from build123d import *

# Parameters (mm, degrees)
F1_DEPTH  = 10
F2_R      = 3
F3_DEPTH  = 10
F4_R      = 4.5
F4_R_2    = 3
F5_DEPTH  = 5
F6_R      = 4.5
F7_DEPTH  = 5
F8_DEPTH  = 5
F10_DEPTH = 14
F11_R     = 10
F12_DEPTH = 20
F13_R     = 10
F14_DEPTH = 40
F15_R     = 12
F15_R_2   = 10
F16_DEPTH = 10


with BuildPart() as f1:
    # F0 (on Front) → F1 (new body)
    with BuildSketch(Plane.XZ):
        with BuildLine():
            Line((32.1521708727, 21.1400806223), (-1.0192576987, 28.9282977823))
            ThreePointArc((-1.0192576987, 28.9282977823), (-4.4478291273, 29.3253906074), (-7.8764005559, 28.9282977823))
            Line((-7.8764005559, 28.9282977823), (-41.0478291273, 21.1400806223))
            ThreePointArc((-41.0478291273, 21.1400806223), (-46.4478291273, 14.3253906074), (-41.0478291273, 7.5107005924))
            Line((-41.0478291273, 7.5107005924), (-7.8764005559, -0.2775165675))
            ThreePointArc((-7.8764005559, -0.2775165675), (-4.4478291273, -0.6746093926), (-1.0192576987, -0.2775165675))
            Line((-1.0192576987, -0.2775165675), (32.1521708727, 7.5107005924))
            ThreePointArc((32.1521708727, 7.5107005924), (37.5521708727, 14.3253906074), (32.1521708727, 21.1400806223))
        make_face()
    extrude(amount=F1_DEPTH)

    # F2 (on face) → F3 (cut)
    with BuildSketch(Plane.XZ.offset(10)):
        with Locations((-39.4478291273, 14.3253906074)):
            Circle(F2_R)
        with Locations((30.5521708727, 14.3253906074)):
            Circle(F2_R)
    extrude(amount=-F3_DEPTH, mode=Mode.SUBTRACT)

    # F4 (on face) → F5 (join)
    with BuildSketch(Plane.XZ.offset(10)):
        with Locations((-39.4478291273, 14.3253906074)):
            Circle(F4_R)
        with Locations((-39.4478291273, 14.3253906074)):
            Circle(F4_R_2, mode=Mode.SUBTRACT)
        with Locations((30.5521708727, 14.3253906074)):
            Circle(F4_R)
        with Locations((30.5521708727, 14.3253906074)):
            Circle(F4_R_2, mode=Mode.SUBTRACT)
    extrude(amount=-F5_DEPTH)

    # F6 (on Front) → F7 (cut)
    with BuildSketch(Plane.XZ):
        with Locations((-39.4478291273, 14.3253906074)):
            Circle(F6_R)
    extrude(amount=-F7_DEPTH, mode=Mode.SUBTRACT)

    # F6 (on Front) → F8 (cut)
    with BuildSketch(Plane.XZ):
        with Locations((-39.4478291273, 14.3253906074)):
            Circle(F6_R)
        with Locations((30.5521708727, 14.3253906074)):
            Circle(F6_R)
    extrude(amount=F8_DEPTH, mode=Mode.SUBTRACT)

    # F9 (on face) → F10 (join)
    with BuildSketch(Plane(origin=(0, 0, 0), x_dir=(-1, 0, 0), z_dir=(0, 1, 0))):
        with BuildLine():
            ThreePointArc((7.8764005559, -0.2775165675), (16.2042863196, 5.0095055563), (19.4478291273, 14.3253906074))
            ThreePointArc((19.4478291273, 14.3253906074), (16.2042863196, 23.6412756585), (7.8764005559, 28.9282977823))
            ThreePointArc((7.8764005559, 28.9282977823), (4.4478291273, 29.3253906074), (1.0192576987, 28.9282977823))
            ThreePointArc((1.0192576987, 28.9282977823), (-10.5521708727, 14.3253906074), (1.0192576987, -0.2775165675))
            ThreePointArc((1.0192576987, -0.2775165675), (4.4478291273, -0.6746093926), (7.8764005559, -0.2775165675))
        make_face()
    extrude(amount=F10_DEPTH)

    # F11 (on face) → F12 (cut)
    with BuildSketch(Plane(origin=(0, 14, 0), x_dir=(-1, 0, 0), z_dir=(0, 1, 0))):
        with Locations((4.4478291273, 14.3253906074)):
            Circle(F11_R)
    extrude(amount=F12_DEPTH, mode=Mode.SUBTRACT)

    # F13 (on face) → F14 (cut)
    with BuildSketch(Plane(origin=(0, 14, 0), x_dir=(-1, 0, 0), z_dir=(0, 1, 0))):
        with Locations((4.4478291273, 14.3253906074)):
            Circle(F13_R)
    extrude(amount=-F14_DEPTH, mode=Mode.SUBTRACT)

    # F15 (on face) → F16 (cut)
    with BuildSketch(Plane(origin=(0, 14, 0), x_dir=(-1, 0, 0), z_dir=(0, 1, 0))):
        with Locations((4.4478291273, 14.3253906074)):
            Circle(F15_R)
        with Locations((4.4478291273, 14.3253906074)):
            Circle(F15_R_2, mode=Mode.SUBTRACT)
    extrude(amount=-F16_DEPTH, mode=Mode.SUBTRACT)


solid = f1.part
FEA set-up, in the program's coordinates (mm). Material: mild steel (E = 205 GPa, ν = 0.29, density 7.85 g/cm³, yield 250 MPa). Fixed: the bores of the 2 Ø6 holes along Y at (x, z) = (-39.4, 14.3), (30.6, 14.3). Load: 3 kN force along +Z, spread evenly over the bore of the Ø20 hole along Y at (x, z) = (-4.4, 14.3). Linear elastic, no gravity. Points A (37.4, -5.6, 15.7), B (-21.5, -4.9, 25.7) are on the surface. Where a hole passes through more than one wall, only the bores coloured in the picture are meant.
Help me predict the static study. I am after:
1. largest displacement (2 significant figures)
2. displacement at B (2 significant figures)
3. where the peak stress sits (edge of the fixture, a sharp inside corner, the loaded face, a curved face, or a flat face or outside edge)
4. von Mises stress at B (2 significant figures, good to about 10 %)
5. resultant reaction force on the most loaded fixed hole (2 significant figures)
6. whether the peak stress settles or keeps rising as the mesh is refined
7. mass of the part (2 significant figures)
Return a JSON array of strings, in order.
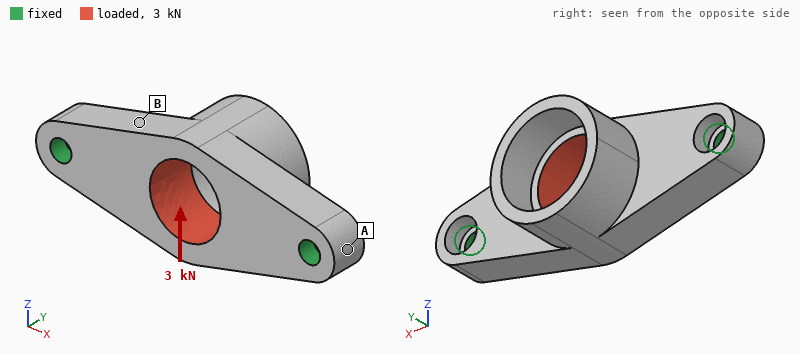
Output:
["19 µm", "8.4 µm", "edge of the fixture", "25 MPa", "1.5 kN", "keeps rising", "140 g"]
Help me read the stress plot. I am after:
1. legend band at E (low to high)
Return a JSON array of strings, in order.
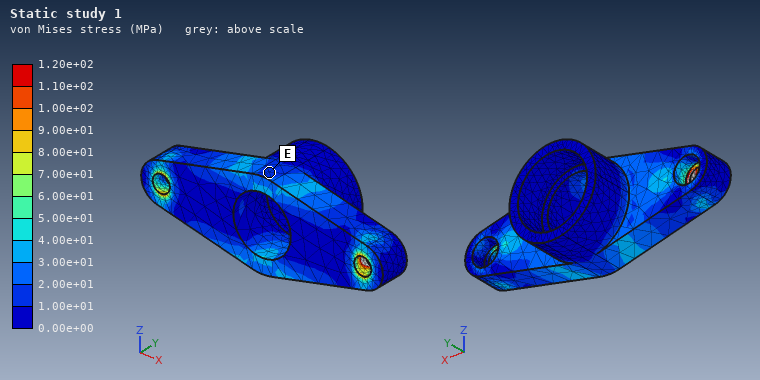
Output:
["1.00e+01 to 2.00e+01 MPa"]
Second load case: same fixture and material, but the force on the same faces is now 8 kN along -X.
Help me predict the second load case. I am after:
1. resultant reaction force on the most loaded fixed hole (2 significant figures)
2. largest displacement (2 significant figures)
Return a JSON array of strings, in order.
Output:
["4.0 kN", "4.4 µm"]
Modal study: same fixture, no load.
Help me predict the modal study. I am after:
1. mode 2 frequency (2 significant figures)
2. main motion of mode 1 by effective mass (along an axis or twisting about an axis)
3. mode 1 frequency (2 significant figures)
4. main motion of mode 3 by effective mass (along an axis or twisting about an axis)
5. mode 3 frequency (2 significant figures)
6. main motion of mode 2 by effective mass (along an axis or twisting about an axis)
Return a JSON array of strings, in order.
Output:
["6700 Hz", "along Z", "5800 Hz", "along Z", "13 kHz", "along Y"]
